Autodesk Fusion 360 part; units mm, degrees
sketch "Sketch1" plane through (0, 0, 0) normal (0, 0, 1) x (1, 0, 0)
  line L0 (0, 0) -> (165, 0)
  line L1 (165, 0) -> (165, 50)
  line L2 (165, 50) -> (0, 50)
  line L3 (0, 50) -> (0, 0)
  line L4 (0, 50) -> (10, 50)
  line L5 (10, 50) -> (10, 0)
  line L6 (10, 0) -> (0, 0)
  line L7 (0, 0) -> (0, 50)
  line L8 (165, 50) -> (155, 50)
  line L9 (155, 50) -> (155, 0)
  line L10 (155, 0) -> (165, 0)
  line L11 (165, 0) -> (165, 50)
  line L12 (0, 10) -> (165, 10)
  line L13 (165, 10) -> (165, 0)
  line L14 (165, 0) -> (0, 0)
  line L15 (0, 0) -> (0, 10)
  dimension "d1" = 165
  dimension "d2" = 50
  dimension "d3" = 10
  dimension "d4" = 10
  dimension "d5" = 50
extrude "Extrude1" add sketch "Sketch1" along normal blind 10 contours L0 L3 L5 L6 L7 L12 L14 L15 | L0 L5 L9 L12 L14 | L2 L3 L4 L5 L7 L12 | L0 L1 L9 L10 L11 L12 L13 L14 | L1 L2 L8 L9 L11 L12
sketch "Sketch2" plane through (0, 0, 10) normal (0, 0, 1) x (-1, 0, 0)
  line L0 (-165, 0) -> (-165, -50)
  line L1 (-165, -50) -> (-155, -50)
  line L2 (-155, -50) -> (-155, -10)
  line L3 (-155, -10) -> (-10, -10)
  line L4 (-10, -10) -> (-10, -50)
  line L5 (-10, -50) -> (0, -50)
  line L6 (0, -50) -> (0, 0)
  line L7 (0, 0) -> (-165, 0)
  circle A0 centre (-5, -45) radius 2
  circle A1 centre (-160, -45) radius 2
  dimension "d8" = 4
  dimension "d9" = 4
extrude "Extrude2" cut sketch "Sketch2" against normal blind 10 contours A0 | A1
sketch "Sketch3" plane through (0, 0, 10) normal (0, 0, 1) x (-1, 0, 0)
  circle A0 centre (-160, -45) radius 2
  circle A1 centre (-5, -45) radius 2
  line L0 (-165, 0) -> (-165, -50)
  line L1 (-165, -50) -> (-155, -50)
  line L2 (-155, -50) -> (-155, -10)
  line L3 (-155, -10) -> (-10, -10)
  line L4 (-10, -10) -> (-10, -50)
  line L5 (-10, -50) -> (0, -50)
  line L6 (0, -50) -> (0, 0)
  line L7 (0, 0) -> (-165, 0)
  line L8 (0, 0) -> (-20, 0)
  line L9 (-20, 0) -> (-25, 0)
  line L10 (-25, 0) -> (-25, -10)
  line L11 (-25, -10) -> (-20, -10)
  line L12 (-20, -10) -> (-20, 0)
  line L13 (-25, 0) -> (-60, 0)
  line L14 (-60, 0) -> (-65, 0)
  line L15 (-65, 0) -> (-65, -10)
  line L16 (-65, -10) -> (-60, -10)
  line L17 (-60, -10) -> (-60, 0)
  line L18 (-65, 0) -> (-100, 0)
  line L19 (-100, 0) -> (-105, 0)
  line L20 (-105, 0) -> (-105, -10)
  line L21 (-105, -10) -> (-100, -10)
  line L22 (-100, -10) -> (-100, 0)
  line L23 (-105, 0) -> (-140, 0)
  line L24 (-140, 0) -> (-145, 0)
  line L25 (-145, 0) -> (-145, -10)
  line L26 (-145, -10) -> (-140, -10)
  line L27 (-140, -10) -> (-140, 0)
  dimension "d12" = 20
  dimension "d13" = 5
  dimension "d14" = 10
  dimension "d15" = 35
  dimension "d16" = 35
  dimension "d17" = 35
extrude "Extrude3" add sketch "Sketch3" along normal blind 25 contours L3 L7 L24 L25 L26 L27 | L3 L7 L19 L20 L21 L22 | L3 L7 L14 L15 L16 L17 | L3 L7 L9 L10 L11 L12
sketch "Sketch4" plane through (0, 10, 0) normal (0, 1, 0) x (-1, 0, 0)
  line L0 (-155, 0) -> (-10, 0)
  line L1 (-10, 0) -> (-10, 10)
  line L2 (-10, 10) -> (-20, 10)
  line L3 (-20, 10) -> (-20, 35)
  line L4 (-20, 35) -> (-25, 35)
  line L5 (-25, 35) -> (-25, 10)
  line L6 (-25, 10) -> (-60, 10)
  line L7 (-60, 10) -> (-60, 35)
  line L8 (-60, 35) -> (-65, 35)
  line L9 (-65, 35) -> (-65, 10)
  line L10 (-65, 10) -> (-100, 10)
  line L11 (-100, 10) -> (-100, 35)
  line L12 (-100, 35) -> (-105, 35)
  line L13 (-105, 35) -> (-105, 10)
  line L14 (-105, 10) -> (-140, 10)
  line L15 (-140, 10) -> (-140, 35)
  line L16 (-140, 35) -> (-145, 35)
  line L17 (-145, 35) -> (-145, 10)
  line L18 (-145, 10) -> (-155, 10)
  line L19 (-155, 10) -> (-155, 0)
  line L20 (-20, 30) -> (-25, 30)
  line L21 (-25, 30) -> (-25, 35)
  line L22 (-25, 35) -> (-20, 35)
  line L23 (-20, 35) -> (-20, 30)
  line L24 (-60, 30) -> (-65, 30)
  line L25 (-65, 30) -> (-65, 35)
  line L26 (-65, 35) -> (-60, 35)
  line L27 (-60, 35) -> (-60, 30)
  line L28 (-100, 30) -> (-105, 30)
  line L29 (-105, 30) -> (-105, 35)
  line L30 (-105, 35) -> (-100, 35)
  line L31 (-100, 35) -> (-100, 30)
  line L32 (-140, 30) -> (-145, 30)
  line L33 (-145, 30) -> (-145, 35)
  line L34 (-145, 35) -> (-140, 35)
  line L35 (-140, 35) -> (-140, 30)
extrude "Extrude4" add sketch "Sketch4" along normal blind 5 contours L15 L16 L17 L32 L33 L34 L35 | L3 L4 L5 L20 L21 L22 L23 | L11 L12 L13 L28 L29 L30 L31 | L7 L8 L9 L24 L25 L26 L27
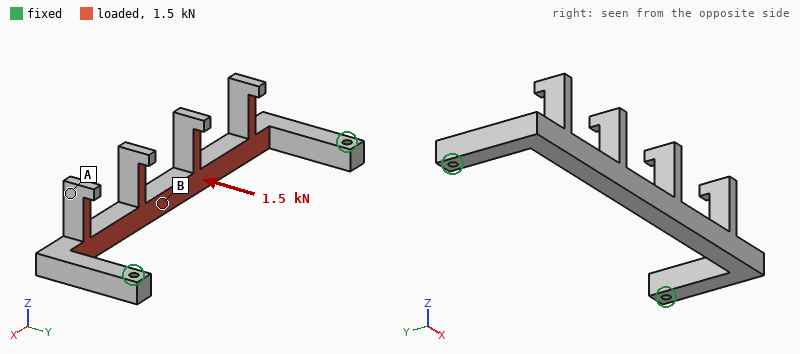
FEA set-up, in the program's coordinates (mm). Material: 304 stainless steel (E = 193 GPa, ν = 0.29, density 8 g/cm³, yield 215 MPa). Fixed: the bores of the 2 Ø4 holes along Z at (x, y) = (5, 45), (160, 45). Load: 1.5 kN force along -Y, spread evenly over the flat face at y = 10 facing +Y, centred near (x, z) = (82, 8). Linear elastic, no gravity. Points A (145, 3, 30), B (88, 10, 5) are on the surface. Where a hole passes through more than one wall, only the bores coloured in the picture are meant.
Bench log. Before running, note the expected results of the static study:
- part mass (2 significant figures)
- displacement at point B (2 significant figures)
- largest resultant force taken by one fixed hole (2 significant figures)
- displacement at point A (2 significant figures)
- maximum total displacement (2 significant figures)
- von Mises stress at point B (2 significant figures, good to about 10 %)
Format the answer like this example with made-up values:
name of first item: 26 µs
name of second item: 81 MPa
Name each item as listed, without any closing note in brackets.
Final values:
part mass: 240 g
displacement at point B: 0.13 mm
largest resultant force taken by one fixed hole: 980 N
displacement at point A: 0.051 mm
maximum total displacement: 0.17 mm
von Mises stress at point B: 64 MPa
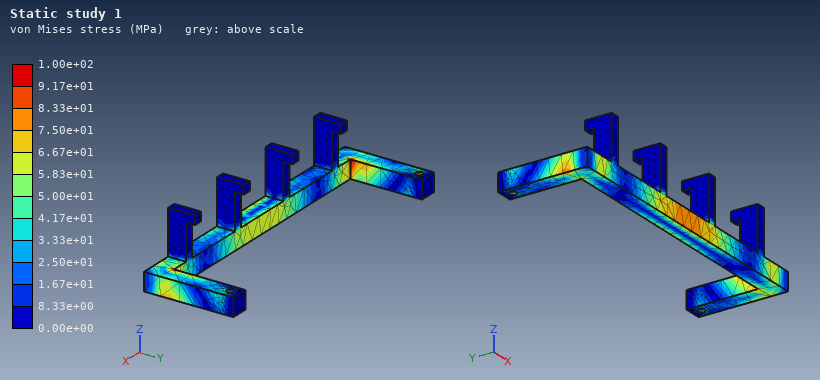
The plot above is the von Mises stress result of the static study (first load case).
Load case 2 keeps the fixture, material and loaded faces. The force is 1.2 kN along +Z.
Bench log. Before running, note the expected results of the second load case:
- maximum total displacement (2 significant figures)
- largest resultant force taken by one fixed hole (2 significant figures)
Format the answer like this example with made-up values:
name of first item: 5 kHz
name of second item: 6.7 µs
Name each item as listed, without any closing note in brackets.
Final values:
maximum total displacement: 0.27 mm
largest resultant force taken by one fixed hole: 600 N
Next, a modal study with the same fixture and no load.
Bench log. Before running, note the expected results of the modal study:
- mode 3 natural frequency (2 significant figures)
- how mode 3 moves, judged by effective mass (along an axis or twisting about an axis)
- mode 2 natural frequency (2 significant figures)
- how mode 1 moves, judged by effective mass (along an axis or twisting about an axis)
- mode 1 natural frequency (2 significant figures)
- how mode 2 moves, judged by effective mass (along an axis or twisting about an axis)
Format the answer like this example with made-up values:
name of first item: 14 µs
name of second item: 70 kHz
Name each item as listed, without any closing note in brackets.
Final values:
mode 3 natural frequency: 1700 Hz
how mode 3 moves, judged by effective mass: along X
mode 2 natural frequency: 1400 Hz
how mode 1 moves, judged by effective mass: along Z
mode 1 natural frequency: 890 Hz
how mode 2 moves, judged by effective mass: along Y
